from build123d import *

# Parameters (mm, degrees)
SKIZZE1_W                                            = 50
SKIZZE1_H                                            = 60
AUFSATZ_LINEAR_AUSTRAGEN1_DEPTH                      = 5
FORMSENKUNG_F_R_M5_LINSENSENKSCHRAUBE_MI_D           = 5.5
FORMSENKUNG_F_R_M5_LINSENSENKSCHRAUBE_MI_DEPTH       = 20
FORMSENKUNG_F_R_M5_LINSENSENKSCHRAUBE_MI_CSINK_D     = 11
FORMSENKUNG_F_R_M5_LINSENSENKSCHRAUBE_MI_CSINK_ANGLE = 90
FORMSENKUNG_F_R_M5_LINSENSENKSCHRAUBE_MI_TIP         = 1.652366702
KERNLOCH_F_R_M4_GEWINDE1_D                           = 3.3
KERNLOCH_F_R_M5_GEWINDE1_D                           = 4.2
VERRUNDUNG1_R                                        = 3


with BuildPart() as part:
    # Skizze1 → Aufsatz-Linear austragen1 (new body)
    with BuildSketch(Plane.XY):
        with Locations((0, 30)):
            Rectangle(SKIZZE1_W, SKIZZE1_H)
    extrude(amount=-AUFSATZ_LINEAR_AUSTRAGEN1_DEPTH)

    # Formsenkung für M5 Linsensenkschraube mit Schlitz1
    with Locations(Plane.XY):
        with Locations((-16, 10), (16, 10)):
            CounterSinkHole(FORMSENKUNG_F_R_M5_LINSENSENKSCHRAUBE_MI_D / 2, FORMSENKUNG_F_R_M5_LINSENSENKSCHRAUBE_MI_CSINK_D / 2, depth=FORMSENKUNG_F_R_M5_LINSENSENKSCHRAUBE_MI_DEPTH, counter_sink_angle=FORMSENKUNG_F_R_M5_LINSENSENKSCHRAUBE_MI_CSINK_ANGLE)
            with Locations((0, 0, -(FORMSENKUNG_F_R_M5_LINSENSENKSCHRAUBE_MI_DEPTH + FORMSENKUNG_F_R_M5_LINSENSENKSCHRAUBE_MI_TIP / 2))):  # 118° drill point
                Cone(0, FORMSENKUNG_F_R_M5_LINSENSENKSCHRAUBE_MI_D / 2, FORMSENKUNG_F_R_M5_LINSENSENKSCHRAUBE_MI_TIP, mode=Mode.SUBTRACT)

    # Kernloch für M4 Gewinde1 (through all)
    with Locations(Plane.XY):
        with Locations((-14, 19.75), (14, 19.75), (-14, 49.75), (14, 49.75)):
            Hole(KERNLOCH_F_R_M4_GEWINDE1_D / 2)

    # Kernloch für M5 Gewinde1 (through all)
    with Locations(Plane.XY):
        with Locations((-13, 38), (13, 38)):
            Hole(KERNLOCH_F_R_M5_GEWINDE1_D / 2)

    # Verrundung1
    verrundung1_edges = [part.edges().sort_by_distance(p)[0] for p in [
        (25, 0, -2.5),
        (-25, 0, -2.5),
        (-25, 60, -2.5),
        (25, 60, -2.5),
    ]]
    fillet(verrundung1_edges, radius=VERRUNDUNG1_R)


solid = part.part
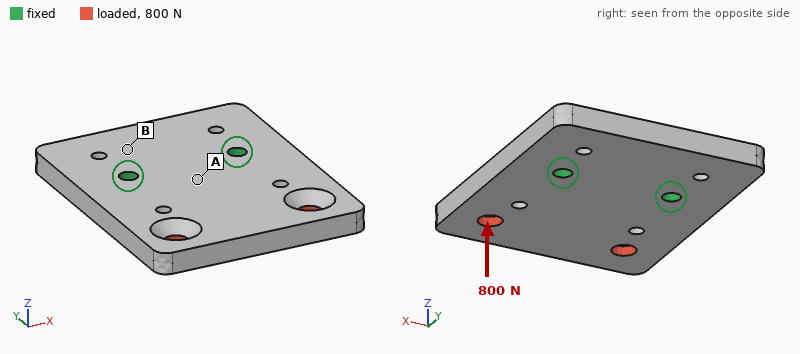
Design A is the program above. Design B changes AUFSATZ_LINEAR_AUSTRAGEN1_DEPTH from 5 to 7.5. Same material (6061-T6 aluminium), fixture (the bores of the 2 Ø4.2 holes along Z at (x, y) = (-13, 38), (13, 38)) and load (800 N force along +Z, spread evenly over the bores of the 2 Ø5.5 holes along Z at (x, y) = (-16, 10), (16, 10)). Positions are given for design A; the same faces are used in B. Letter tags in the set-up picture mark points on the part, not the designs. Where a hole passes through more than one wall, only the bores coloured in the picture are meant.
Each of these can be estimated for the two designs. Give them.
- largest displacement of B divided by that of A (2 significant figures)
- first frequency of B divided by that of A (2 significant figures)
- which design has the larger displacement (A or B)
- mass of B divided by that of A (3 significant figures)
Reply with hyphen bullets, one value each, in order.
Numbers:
- 0.33
- 1.4
- A
- 1.51
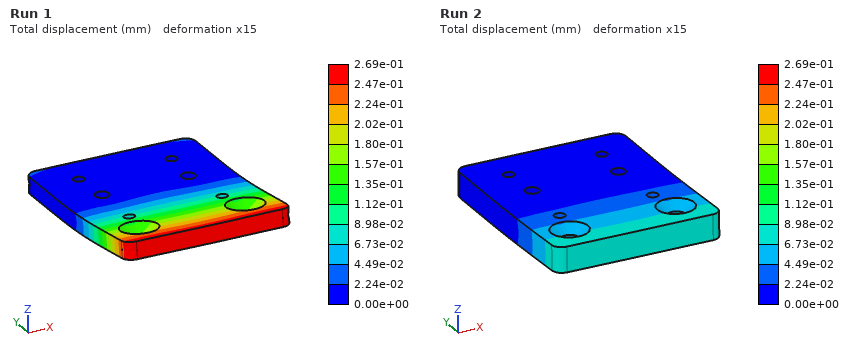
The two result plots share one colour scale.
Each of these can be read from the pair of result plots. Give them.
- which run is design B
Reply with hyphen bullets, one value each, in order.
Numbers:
- Run 2
